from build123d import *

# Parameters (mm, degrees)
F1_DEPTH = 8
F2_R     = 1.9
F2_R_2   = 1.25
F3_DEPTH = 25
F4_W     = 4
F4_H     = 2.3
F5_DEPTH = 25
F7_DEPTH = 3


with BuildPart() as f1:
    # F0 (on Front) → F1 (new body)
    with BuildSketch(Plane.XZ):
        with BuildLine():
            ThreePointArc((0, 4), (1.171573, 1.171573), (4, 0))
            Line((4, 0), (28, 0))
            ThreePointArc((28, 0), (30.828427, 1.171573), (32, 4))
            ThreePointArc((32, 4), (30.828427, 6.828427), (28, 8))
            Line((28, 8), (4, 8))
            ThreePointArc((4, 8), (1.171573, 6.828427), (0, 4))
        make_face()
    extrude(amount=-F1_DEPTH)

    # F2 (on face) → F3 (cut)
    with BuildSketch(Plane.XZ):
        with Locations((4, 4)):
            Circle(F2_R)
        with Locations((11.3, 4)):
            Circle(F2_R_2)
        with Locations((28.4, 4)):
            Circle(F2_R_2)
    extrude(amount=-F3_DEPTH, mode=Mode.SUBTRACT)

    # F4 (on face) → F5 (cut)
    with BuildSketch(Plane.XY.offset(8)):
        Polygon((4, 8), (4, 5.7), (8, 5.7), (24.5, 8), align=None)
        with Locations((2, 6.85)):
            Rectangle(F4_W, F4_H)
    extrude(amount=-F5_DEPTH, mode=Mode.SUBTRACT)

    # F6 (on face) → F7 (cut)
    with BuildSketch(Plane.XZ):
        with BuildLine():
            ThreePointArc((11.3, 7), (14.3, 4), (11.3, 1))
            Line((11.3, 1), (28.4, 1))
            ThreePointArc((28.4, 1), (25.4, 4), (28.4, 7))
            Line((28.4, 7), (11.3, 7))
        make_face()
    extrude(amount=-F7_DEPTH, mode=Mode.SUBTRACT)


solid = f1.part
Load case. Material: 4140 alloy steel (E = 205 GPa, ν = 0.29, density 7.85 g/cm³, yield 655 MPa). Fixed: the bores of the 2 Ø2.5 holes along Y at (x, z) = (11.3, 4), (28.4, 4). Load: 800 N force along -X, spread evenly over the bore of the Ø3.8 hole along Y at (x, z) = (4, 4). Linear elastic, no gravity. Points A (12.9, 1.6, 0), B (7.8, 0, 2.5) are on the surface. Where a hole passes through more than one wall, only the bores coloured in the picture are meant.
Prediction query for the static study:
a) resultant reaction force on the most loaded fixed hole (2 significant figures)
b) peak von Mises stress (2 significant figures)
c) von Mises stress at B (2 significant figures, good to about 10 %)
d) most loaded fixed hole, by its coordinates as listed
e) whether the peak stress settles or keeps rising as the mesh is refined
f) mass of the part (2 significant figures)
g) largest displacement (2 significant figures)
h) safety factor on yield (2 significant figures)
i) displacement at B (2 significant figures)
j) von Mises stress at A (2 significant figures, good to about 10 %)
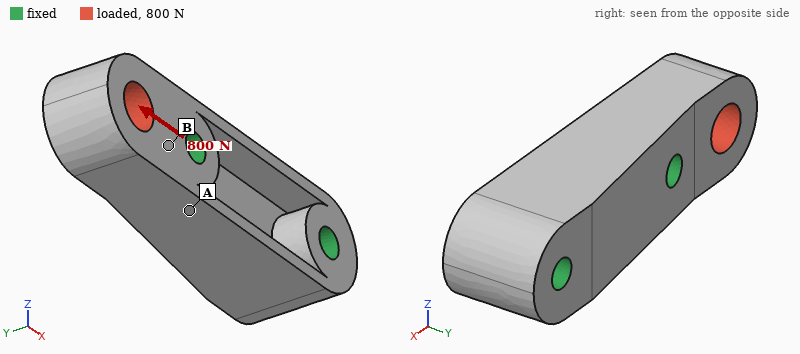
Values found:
750 N
52 MPa
21 MPa
(11.3, 4)
settles
10 g
1.4 µm
13
0.34 µm
7.3 MPa
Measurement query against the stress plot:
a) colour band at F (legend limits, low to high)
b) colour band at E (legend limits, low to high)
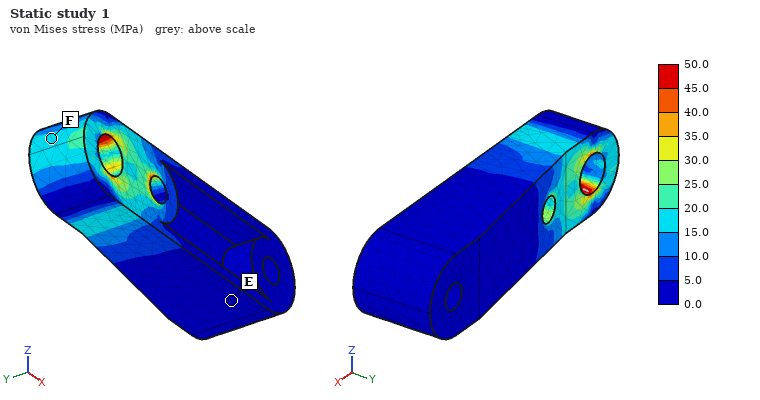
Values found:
15.0 to 20.0 MPa
0.0 to 5.0 MPa
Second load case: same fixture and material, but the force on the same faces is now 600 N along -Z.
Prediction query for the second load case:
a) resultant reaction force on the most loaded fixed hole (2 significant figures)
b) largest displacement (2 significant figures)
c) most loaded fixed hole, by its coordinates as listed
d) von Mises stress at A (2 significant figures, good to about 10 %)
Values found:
700 N
7.8 µm
(11.3, 4)
34 MPa
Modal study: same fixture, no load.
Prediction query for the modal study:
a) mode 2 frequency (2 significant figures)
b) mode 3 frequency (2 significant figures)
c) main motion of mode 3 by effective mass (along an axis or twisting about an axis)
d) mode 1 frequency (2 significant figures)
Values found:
39 kHz
56 kHz
along Z
36 kHz
